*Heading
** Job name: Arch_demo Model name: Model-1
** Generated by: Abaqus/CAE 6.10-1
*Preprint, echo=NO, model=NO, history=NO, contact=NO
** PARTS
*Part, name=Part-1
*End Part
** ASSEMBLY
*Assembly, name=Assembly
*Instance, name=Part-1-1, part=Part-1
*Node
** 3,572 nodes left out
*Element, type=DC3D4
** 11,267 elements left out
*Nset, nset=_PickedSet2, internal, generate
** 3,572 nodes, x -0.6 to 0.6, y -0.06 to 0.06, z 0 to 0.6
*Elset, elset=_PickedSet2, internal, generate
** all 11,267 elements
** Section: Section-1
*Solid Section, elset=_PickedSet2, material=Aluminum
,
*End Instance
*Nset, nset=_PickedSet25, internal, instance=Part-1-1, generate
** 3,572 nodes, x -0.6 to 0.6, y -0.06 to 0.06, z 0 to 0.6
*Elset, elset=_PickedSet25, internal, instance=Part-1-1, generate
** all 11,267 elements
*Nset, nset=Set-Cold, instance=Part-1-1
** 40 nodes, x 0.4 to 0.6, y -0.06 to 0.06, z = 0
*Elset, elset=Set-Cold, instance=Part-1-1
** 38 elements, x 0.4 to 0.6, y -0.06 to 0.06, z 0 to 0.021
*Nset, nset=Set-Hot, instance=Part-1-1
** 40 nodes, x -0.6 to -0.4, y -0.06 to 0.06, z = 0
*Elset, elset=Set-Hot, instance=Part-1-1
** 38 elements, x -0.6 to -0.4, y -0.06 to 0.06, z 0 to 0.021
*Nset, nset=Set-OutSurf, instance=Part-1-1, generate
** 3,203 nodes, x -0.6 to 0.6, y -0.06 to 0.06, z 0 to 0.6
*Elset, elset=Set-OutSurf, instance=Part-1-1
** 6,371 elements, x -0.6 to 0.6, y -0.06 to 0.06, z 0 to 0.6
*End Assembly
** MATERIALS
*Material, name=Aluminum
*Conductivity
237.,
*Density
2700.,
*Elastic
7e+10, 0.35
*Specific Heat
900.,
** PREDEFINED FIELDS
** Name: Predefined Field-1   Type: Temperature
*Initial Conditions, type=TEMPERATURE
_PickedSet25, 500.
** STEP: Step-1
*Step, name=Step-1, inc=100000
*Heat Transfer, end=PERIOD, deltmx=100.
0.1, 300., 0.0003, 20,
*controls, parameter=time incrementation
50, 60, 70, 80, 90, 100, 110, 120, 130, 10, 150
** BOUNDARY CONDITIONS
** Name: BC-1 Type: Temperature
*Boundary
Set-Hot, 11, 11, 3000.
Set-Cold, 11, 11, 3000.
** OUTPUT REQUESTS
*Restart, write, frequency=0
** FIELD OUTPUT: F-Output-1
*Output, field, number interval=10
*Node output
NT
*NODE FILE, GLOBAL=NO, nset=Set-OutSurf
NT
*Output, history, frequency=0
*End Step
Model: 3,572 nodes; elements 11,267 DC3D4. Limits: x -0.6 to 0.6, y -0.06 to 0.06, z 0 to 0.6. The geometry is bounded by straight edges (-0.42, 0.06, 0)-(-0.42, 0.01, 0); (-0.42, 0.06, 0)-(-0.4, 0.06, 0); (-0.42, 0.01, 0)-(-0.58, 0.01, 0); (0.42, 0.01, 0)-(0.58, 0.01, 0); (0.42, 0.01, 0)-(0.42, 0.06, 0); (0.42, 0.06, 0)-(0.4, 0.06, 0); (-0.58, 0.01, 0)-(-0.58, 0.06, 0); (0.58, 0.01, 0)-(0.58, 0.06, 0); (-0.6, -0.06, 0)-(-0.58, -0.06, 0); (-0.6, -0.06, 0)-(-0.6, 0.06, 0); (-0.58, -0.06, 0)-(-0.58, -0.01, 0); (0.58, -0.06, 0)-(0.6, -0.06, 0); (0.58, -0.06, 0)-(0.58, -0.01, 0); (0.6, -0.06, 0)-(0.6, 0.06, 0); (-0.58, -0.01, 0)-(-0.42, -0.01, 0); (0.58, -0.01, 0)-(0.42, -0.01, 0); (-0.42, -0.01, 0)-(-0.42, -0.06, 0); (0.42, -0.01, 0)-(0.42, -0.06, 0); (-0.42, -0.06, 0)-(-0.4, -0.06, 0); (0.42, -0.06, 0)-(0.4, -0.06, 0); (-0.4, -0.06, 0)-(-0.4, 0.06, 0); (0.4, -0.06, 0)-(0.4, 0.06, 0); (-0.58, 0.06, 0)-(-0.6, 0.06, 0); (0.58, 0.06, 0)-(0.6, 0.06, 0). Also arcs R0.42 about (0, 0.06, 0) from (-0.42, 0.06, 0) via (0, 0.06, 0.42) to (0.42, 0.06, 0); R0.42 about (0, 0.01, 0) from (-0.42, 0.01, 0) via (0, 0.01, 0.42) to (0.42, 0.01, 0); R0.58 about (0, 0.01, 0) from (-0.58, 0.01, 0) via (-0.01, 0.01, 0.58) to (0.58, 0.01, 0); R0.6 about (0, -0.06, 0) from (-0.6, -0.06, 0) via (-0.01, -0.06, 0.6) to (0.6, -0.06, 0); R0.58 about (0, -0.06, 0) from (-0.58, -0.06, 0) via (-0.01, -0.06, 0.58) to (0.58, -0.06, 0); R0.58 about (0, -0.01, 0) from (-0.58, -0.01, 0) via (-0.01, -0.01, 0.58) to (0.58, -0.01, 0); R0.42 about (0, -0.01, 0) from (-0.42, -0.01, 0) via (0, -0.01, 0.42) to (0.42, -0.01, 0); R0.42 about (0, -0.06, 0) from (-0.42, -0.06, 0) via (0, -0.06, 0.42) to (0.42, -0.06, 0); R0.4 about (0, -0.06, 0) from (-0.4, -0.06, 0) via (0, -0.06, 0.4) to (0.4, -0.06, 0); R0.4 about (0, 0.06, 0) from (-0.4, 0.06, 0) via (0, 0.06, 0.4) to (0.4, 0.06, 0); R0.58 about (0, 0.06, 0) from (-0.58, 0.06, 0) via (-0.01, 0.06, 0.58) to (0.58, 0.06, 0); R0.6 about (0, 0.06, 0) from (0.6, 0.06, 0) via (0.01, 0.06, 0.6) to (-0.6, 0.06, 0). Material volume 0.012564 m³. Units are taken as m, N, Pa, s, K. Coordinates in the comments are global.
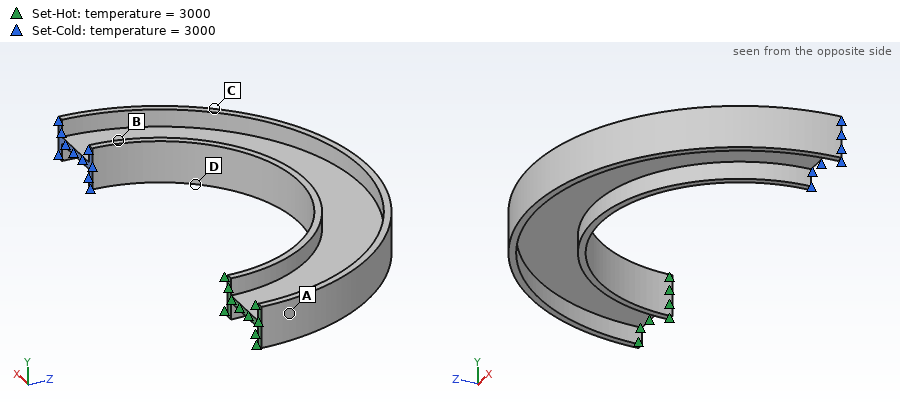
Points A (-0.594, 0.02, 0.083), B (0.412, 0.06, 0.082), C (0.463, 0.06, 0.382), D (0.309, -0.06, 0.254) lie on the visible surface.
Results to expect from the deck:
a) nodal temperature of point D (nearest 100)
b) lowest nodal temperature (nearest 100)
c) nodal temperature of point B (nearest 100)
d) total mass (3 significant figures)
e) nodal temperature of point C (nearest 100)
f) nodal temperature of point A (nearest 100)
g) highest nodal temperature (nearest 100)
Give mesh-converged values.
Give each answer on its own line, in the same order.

1000 K
500 K
2300 K
33.9 kg
800 K
2400 K
3000 K
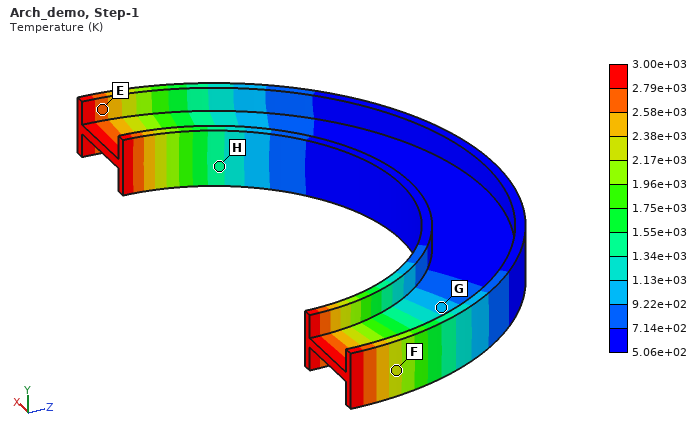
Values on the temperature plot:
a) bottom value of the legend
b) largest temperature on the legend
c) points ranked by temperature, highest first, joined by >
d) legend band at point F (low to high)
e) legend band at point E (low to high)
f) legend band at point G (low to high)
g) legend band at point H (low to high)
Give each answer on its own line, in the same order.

5.06e+02 K
3.00e+03 K
E > F > H > G
2.17e+03 to 2.38e+03 K
2.58e+03 to 2.79e+03 K
9.22e+02 to 1.13e+03 K
1.34e+03 to 1.55e+03 K
